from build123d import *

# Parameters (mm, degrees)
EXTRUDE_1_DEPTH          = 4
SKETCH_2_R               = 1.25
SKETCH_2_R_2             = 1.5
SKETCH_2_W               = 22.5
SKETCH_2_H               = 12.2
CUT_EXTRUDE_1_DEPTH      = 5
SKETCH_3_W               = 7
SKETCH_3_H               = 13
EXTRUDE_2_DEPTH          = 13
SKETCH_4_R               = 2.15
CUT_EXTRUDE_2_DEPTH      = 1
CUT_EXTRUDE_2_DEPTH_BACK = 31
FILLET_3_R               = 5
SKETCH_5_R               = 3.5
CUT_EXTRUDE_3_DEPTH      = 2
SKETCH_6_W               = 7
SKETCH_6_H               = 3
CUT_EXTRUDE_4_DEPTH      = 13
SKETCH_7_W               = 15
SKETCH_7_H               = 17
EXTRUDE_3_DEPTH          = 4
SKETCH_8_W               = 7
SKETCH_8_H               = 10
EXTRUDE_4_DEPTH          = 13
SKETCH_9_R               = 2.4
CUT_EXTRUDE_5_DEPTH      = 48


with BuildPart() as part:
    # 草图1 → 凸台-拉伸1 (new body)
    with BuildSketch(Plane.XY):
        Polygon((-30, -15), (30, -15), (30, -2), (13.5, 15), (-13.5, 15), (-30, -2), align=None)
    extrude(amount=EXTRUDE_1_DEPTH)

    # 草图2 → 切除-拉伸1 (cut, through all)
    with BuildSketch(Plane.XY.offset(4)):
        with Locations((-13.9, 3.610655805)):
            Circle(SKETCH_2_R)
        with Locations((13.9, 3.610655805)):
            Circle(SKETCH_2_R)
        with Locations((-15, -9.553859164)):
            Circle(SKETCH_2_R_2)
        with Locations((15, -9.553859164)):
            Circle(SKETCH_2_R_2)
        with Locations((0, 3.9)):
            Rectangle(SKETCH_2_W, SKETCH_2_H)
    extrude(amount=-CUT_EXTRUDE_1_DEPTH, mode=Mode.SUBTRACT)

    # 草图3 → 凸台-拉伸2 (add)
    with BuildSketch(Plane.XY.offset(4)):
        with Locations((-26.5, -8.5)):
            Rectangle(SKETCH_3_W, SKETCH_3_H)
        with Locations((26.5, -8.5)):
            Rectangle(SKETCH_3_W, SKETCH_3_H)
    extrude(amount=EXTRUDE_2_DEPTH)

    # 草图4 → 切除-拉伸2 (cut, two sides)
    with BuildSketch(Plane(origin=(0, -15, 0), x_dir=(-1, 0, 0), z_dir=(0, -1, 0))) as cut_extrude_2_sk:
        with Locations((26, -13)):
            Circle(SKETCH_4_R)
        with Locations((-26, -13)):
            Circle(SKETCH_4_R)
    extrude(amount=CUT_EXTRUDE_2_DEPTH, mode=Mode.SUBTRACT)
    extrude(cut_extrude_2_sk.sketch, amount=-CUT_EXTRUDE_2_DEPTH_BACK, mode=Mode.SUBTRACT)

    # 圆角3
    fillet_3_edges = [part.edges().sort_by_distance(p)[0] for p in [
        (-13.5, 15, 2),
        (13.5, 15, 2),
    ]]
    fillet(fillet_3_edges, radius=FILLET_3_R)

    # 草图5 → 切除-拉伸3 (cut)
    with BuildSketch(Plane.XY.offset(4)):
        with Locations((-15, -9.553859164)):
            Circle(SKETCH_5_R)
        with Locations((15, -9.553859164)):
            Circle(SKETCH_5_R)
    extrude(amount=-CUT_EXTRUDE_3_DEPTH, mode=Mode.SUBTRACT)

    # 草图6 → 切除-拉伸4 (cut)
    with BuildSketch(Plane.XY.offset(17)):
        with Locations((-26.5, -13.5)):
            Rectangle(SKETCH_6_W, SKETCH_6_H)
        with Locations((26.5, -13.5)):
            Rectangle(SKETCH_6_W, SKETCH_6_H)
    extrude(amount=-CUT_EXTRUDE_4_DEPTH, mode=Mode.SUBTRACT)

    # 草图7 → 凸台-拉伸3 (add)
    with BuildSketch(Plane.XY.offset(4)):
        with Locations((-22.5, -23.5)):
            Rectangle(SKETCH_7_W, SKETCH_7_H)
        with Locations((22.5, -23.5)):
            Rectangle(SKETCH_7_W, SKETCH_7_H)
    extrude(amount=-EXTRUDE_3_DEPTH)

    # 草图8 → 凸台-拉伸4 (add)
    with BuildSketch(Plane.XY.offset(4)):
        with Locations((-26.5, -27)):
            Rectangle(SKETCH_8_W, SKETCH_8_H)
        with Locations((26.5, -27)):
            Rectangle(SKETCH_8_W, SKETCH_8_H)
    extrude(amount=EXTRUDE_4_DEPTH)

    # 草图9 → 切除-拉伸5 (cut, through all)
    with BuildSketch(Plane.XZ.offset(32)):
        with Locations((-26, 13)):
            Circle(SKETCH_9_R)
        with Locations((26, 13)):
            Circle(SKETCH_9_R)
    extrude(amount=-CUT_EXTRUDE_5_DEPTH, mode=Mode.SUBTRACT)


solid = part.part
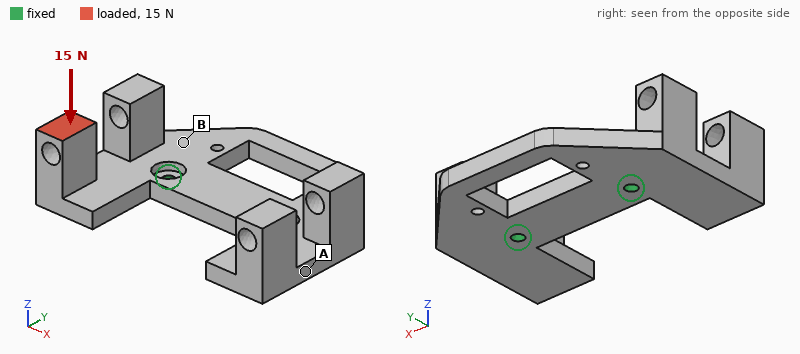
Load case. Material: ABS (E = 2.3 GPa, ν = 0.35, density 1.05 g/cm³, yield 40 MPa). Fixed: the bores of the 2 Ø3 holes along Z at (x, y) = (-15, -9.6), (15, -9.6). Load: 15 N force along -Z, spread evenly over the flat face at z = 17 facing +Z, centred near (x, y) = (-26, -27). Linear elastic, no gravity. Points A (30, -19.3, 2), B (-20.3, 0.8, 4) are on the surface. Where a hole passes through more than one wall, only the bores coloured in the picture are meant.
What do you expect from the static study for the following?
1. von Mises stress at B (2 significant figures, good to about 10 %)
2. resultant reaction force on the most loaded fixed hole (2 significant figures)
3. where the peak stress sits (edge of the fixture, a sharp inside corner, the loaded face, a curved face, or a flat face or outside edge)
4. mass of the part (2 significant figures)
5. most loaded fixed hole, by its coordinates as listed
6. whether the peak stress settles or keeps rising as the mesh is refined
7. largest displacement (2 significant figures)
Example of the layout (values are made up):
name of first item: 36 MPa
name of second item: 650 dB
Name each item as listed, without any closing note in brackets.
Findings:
von Mises stress at B: 2.1 MPa
resultant reaction force on the most loaded fixed hole: 22 N
where the peak stress sits: edge of the fixture
mass of the part: 10 g
most loaded fixed hole, by its coordinates as listed: (-15, -9.6)
whether the peak stress settles or keeps rising as the mesh is refined: keeps rising
largest displacement: 0.71 mm
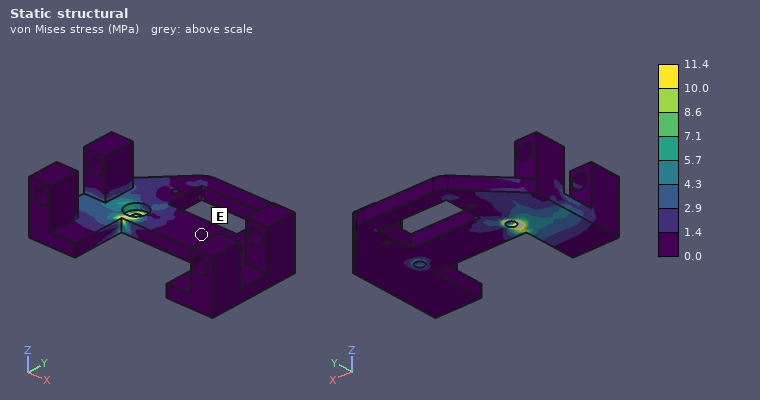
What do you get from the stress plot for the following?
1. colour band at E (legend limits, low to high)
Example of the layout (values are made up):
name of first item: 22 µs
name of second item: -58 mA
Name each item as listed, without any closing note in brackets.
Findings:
colour band at E: 0.0 to 1.4 MPa
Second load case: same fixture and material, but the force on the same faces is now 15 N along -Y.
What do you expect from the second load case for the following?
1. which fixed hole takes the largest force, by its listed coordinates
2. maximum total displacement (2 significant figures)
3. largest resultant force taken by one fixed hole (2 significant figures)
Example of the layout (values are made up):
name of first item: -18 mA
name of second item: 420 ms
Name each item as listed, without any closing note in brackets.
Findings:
which fixed hole takes the largest force, by its listed coordinates: (-15, -9.6)
maximum total displacement: 0.71 mm
largest resultant force taken by one fixed hole: 19 N
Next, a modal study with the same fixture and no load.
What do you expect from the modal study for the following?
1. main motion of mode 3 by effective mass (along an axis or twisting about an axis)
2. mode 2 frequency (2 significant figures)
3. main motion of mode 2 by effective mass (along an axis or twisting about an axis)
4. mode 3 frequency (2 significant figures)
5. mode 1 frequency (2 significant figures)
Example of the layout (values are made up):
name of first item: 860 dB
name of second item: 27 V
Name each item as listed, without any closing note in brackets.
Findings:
main motion of mode 3 by effective mass: along Z
mode 2 frequency: 740 Hz
main motion of mode 2 by effective mass: twisting about Y
mode 3 frequency: 1100 Hz
mode 1 frequency: 620 Hz
